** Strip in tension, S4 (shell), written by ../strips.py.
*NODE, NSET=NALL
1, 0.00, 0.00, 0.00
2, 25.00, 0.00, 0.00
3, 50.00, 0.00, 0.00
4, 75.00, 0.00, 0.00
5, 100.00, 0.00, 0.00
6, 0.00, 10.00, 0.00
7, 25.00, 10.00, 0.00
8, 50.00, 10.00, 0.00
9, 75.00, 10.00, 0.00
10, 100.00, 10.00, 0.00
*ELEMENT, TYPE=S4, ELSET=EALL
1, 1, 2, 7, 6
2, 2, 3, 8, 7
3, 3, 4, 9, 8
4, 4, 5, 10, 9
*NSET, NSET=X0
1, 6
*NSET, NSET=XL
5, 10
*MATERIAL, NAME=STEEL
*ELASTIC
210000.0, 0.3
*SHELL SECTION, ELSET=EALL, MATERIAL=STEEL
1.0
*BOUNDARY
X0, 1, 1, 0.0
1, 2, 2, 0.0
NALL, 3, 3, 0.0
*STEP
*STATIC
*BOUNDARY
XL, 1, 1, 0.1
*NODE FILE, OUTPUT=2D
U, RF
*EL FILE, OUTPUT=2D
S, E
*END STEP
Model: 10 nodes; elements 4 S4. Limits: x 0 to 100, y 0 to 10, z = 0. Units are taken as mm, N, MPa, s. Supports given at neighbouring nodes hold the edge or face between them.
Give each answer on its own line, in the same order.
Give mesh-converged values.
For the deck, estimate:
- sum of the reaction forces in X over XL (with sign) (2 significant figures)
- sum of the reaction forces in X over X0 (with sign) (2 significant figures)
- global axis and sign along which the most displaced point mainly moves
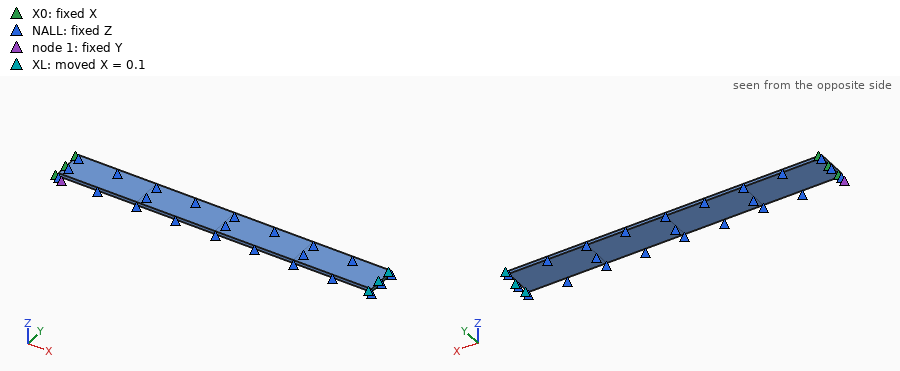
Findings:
2100 N
-2100 N
+X
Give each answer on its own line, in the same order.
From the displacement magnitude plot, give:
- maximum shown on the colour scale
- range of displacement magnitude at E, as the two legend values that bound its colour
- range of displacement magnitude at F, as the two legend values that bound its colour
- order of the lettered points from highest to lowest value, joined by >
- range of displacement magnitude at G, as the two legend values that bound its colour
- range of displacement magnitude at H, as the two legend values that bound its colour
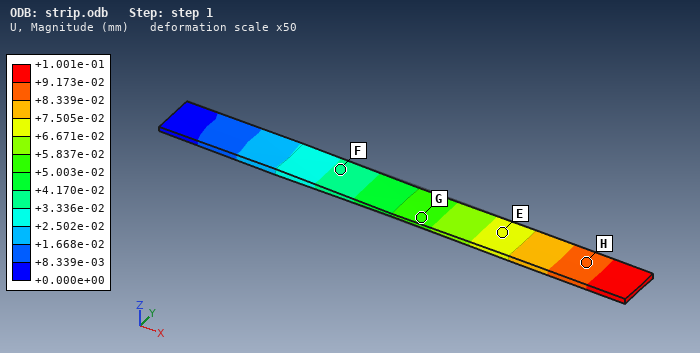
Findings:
+1.001e-01 mm
+6.671e-02 to +7.505e-02 mm
+3.336e-02 to +4.170e-02 mm
H > E > G > F
+5.003e-02 to +5.837e-02 mm
+8.339e-02 to +9.173e-02 mm
